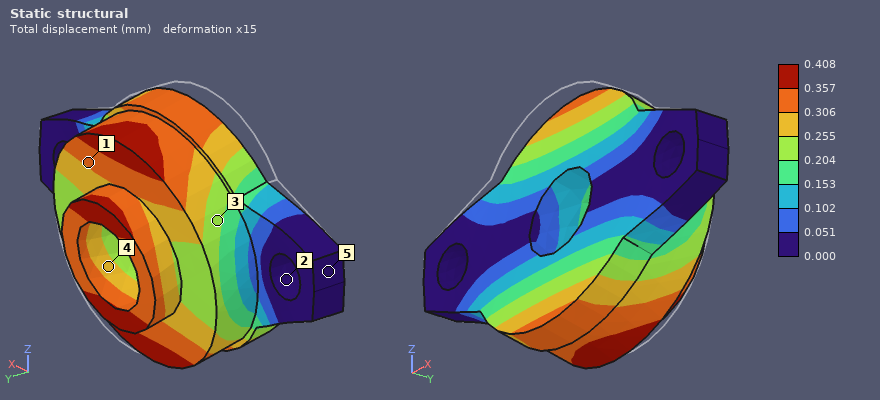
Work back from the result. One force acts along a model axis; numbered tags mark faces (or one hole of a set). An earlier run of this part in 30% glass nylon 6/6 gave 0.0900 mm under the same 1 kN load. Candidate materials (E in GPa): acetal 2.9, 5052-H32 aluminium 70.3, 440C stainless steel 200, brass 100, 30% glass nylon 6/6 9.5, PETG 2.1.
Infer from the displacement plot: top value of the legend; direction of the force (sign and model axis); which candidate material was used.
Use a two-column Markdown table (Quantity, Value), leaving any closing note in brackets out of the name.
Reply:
| Quantity | Value |
|---|---|
| top value of the legend | 0.408 mm |
| direction of the force | -Z |
| which candidate material was used | PETG |
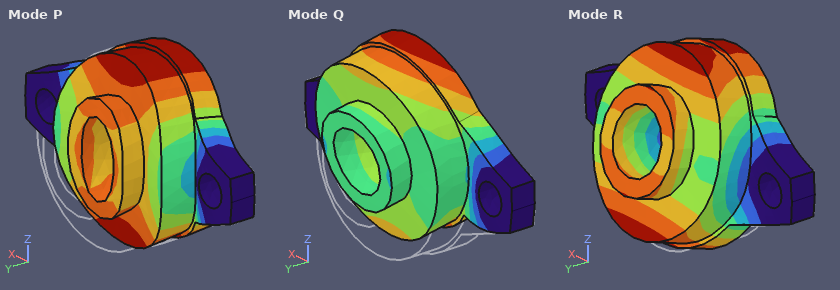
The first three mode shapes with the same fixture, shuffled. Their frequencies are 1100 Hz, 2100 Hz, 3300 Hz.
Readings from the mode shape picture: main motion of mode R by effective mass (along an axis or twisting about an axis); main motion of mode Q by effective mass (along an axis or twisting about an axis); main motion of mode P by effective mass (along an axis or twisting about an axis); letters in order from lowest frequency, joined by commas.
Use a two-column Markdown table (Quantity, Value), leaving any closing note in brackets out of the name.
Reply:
| Quantity | Value |
|---|---|
| main motion of mode R by effective mass | along Z |
| main motion of mode Q by effective mass | along Z |
| main motion of mode P by effective mass | along Y |
| letters in order from lowest frequency, joined by commas | R, P, Q |
